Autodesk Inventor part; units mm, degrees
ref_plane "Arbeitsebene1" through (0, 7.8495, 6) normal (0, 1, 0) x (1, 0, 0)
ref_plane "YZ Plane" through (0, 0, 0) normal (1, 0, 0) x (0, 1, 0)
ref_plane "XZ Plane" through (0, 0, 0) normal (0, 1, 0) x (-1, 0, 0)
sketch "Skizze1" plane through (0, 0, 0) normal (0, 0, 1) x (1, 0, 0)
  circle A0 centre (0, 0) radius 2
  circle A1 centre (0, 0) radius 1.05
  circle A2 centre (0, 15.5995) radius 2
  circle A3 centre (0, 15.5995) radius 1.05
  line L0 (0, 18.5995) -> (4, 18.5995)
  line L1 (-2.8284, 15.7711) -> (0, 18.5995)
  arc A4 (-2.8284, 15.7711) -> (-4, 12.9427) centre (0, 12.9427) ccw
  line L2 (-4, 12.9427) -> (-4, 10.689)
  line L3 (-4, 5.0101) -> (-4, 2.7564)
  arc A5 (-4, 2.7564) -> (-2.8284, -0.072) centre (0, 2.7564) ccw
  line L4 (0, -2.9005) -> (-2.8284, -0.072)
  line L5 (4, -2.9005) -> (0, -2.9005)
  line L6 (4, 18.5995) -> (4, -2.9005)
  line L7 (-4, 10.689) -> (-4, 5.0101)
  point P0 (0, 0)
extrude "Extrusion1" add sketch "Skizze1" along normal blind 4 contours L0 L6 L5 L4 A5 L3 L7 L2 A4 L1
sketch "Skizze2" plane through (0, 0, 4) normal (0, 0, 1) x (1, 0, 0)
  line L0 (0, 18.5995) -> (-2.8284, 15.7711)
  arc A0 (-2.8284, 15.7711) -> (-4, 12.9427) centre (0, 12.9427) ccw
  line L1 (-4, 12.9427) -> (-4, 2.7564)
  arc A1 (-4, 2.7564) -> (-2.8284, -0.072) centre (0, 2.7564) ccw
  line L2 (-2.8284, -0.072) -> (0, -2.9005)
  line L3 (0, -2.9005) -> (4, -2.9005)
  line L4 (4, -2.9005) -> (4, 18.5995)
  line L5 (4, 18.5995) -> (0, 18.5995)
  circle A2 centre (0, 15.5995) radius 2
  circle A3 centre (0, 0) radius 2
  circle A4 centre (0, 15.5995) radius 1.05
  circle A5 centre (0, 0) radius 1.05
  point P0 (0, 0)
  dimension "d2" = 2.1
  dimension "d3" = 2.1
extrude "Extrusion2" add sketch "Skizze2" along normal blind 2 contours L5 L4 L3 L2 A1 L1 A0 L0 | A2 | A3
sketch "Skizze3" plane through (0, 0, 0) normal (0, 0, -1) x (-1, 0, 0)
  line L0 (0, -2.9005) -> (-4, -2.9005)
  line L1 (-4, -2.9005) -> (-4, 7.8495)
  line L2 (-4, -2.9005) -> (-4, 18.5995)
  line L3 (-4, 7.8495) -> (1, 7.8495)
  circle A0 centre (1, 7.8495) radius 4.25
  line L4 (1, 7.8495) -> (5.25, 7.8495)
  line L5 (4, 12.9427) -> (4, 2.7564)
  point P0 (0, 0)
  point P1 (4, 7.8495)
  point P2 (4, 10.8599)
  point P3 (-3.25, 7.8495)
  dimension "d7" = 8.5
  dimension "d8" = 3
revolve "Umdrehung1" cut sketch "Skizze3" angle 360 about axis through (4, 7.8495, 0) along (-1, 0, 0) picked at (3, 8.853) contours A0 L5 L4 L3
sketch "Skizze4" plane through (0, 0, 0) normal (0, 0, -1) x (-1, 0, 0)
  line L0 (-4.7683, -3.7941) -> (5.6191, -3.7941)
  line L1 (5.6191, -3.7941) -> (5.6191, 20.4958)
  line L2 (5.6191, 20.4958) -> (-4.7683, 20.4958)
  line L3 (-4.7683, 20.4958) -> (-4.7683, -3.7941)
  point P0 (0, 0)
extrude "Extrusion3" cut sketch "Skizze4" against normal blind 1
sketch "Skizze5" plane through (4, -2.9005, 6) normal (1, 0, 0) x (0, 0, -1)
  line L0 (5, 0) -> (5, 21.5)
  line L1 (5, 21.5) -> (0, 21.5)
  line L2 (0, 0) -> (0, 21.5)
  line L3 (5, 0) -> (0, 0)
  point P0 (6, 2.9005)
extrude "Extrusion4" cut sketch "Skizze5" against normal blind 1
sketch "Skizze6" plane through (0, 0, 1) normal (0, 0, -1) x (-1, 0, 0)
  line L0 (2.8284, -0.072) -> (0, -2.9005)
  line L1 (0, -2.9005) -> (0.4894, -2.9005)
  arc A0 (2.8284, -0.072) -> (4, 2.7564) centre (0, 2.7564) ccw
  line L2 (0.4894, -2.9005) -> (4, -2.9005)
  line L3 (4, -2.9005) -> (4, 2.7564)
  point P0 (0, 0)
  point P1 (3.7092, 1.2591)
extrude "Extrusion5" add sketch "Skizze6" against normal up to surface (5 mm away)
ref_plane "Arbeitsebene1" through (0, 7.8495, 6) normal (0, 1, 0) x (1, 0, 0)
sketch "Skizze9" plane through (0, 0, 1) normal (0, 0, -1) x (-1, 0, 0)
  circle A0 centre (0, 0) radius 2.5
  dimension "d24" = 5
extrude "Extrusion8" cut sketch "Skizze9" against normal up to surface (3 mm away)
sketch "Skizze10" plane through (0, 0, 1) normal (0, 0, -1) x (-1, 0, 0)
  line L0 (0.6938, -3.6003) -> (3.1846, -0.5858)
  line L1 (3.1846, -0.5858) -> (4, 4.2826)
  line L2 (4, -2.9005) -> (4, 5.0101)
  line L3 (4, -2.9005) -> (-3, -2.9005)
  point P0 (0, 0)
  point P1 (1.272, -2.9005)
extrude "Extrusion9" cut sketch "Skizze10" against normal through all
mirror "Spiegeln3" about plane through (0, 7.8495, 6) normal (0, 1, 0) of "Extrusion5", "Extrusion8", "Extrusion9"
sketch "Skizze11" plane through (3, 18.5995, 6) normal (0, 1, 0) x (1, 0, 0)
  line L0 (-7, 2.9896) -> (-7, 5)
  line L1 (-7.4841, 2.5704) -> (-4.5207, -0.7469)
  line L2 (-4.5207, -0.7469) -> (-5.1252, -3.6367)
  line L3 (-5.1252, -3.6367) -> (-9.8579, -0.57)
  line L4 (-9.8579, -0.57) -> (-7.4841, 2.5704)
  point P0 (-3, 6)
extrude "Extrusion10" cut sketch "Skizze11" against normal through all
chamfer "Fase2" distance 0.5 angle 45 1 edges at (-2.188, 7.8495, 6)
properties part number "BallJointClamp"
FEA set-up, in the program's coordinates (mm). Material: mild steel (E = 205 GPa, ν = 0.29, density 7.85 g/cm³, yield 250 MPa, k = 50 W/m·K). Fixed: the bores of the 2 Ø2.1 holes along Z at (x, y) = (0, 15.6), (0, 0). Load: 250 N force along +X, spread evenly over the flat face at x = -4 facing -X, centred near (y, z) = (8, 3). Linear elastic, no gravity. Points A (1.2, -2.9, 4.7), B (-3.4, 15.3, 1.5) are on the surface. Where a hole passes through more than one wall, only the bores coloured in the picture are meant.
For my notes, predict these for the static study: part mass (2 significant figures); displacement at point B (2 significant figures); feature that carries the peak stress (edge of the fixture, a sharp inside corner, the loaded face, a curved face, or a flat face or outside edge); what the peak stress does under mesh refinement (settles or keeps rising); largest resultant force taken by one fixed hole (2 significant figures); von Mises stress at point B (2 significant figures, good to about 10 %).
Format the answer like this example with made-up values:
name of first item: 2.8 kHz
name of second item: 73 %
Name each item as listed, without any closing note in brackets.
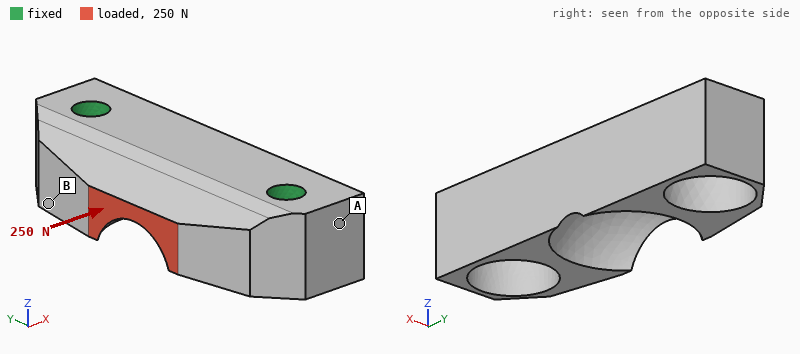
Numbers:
part mass: 3.4 g
displacement at point B: 1.4 µm
feature that carries the peak stress: edge of the fixture
what the peak stress does under mesh refinement: keeps rising
largest resultant force taken by one fixed hole: 130 N
von Mises stress at point B: 19 MPa
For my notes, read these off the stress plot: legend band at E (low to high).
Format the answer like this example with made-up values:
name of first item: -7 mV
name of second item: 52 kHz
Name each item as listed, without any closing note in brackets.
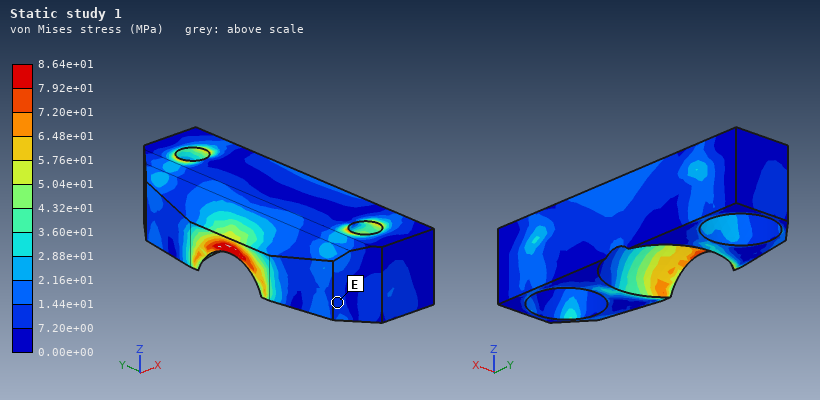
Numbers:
legend band at E: 7.20e+00 to 1.44e+01 MPa
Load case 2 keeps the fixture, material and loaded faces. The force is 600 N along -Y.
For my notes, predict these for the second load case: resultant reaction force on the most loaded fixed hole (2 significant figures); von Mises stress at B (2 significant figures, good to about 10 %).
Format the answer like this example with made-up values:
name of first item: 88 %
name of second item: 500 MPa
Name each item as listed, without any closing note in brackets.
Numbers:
resultant reaction force on the most loaded fixed hole: 340 N
von Mises stress at B: 30 MPa
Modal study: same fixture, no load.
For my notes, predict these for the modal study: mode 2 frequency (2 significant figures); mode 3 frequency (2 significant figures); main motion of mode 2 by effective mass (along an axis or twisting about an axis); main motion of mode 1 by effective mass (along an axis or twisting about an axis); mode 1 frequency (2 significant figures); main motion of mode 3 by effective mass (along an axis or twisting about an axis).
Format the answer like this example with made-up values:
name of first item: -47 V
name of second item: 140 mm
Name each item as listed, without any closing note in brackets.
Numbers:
mode 2 frequency: 45 kHz
mode 3 frequency: 66 kHz
main motion of mode 2 by effective mass: along X
main motion of mode 1 by effective mass: along Z
mode 1 frequency: 42 kHz
main motion of mode 3 by effective mass: along X
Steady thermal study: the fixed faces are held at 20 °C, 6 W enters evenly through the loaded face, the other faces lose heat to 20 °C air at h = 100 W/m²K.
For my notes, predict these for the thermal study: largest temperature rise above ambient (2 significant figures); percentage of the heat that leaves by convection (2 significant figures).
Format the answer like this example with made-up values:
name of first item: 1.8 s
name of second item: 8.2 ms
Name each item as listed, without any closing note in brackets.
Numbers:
largest temperature rise above ambient: 41 K
percentage of the heat that leaves by convection: 8.6 %
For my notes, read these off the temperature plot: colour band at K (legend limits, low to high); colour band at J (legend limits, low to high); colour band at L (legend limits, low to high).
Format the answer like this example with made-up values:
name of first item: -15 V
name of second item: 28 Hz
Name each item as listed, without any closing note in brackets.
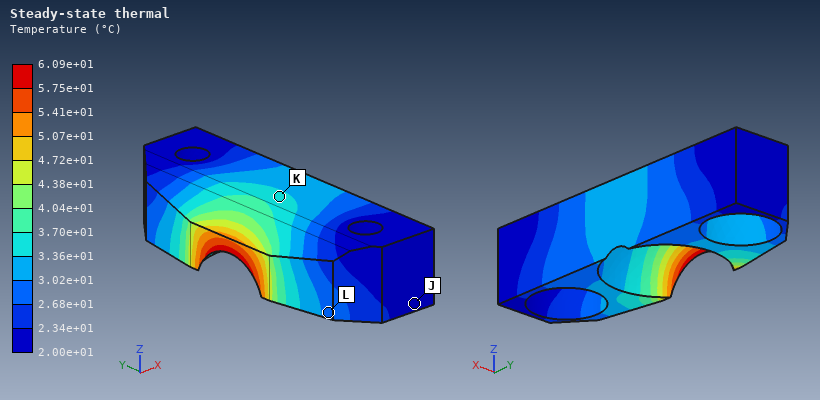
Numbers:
colour band at K: 3.36e+01 to 3.70e+01 °C
colour band at J: 2.00e+01 to 2.34e+01 °C
colour band at L: 2.68e+01 to 3.02e+01 °C
